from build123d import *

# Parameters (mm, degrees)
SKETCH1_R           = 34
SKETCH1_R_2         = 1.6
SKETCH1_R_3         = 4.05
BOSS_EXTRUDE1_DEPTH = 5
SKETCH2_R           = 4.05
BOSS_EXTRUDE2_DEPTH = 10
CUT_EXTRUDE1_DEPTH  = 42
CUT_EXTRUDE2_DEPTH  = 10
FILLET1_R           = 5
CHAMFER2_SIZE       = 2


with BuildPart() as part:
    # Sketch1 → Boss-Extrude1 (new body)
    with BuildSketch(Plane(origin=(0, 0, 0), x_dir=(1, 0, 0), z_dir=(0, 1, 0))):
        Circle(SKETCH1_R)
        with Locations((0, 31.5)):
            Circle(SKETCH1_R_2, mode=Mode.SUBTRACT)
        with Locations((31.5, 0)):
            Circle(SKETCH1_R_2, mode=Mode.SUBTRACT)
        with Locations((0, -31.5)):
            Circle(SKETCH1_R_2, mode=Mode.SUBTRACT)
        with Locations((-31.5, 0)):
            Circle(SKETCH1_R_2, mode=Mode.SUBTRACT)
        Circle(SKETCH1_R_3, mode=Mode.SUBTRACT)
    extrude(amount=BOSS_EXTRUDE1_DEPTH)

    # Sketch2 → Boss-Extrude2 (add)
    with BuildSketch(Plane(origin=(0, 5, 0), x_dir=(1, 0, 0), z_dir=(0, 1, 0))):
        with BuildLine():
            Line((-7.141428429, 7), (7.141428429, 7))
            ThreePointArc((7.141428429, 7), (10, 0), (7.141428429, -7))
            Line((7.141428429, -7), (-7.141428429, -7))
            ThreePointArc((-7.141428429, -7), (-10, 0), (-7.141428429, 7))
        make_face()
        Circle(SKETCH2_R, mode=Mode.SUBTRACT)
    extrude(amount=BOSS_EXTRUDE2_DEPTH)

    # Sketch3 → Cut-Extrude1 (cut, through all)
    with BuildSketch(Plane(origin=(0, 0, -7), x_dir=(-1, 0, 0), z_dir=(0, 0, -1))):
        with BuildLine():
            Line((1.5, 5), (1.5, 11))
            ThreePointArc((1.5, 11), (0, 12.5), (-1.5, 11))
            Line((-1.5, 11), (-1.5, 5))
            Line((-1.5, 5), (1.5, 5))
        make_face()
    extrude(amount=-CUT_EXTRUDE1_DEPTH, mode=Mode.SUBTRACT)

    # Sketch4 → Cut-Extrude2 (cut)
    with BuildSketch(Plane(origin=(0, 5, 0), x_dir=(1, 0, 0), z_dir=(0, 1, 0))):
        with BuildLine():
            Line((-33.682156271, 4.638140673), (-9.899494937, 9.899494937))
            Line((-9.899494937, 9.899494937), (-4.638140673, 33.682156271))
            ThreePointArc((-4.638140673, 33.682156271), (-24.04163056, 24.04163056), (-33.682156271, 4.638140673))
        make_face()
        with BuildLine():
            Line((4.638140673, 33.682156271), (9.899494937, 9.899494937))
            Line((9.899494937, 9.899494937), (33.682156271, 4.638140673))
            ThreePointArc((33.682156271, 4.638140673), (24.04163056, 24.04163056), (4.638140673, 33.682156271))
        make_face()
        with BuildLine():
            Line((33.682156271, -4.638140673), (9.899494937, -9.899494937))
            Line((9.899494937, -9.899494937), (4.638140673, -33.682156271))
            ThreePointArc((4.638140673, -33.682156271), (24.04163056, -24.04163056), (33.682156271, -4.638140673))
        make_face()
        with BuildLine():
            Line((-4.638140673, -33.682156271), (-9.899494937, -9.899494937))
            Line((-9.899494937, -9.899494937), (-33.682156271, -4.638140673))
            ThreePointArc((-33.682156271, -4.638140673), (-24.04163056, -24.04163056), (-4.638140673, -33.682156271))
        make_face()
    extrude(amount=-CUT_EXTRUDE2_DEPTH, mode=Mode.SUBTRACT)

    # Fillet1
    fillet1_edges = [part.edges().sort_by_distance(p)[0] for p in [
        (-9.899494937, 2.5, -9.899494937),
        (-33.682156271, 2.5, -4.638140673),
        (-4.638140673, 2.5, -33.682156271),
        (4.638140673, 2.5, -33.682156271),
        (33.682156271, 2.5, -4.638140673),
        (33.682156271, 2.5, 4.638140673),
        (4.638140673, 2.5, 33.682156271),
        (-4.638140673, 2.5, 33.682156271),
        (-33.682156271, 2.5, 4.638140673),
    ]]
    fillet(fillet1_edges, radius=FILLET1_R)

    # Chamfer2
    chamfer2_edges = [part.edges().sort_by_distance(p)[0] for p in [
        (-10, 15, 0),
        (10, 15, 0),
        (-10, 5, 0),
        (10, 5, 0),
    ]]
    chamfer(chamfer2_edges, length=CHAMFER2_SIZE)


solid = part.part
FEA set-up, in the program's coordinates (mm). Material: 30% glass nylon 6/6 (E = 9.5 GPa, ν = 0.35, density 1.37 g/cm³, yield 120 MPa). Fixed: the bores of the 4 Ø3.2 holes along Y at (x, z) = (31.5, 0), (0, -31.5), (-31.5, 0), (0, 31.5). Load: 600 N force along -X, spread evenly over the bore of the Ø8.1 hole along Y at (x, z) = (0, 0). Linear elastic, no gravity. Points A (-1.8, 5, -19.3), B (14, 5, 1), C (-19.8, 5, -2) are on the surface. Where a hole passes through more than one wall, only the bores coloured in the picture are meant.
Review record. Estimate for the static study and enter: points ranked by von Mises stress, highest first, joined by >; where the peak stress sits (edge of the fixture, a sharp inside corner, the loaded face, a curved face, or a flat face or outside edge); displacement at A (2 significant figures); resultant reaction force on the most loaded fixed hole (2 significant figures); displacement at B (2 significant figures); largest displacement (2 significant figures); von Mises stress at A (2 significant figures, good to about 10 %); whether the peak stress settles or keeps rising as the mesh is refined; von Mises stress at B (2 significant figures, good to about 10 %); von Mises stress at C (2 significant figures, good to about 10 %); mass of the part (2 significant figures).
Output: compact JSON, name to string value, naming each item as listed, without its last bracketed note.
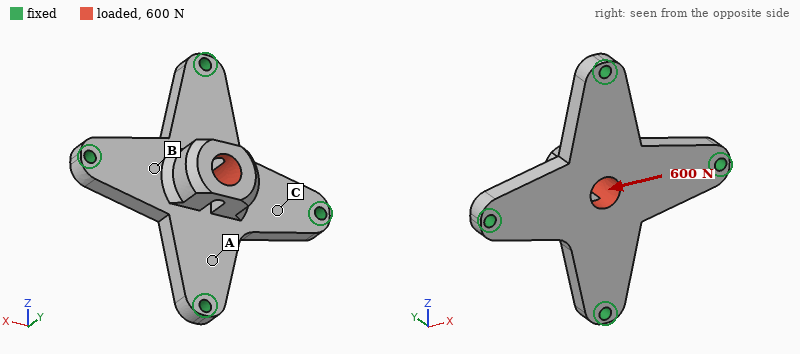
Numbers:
{"points ranked by von Mises stress, highest first, joined by >": "B > C > A", "where the peak stress sits": "edge of the fixture", "displacement at A": "8.9 µm", "resultant reaction force on the most loaded fixed hole": "280 N", "displacement at B": "22 µm", "largest displacement": "43 µm", "von Mises stress at A": "2.8 MPa", "whether the peak stress settles or keeps rising as the mesh is refined": "keeps rising", "von Mises stress at B": "11 MPa", "von Mises stress at C": "7.2 MPa", "mass of the part": "14 g"}
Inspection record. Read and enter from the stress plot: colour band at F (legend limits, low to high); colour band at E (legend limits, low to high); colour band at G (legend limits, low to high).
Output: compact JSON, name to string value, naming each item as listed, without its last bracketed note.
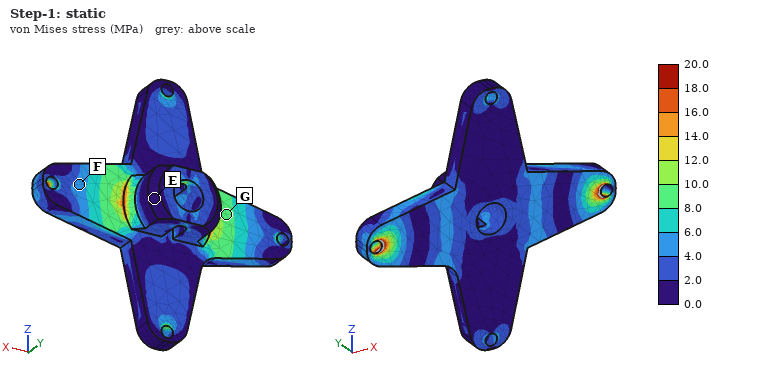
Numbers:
{"colour band at F": "4.0 to 6.0 MPa", "colour band at E": "0.0 to 2.0 MPa", "colour band at G": "8.0 to 10.0 MPa"}
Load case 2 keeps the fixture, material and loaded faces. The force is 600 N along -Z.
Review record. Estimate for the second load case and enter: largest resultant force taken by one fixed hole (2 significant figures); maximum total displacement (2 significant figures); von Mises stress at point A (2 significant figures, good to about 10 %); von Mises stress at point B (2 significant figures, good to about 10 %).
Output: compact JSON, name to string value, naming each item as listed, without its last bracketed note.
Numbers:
{"largest resultant force taken by one fixed hole": "280 N", "maximum total displacement": "60 µm", "von Mises stress at point A": "6.9 MPa", "von Mises stress at point B": "2.8 MPa"}
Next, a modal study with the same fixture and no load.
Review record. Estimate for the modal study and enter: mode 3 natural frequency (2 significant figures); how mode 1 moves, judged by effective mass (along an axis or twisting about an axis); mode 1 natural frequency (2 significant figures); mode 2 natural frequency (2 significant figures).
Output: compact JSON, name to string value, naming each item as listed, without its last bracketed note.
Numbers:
{"mode 3 natural frequency": "7000 Hz", "how mode 1 moves, judged by effective mass": "along Y", "mode 1 natural frequency": "3600 Hz", "mode 2 natural frequency": "6600 Hz"}
